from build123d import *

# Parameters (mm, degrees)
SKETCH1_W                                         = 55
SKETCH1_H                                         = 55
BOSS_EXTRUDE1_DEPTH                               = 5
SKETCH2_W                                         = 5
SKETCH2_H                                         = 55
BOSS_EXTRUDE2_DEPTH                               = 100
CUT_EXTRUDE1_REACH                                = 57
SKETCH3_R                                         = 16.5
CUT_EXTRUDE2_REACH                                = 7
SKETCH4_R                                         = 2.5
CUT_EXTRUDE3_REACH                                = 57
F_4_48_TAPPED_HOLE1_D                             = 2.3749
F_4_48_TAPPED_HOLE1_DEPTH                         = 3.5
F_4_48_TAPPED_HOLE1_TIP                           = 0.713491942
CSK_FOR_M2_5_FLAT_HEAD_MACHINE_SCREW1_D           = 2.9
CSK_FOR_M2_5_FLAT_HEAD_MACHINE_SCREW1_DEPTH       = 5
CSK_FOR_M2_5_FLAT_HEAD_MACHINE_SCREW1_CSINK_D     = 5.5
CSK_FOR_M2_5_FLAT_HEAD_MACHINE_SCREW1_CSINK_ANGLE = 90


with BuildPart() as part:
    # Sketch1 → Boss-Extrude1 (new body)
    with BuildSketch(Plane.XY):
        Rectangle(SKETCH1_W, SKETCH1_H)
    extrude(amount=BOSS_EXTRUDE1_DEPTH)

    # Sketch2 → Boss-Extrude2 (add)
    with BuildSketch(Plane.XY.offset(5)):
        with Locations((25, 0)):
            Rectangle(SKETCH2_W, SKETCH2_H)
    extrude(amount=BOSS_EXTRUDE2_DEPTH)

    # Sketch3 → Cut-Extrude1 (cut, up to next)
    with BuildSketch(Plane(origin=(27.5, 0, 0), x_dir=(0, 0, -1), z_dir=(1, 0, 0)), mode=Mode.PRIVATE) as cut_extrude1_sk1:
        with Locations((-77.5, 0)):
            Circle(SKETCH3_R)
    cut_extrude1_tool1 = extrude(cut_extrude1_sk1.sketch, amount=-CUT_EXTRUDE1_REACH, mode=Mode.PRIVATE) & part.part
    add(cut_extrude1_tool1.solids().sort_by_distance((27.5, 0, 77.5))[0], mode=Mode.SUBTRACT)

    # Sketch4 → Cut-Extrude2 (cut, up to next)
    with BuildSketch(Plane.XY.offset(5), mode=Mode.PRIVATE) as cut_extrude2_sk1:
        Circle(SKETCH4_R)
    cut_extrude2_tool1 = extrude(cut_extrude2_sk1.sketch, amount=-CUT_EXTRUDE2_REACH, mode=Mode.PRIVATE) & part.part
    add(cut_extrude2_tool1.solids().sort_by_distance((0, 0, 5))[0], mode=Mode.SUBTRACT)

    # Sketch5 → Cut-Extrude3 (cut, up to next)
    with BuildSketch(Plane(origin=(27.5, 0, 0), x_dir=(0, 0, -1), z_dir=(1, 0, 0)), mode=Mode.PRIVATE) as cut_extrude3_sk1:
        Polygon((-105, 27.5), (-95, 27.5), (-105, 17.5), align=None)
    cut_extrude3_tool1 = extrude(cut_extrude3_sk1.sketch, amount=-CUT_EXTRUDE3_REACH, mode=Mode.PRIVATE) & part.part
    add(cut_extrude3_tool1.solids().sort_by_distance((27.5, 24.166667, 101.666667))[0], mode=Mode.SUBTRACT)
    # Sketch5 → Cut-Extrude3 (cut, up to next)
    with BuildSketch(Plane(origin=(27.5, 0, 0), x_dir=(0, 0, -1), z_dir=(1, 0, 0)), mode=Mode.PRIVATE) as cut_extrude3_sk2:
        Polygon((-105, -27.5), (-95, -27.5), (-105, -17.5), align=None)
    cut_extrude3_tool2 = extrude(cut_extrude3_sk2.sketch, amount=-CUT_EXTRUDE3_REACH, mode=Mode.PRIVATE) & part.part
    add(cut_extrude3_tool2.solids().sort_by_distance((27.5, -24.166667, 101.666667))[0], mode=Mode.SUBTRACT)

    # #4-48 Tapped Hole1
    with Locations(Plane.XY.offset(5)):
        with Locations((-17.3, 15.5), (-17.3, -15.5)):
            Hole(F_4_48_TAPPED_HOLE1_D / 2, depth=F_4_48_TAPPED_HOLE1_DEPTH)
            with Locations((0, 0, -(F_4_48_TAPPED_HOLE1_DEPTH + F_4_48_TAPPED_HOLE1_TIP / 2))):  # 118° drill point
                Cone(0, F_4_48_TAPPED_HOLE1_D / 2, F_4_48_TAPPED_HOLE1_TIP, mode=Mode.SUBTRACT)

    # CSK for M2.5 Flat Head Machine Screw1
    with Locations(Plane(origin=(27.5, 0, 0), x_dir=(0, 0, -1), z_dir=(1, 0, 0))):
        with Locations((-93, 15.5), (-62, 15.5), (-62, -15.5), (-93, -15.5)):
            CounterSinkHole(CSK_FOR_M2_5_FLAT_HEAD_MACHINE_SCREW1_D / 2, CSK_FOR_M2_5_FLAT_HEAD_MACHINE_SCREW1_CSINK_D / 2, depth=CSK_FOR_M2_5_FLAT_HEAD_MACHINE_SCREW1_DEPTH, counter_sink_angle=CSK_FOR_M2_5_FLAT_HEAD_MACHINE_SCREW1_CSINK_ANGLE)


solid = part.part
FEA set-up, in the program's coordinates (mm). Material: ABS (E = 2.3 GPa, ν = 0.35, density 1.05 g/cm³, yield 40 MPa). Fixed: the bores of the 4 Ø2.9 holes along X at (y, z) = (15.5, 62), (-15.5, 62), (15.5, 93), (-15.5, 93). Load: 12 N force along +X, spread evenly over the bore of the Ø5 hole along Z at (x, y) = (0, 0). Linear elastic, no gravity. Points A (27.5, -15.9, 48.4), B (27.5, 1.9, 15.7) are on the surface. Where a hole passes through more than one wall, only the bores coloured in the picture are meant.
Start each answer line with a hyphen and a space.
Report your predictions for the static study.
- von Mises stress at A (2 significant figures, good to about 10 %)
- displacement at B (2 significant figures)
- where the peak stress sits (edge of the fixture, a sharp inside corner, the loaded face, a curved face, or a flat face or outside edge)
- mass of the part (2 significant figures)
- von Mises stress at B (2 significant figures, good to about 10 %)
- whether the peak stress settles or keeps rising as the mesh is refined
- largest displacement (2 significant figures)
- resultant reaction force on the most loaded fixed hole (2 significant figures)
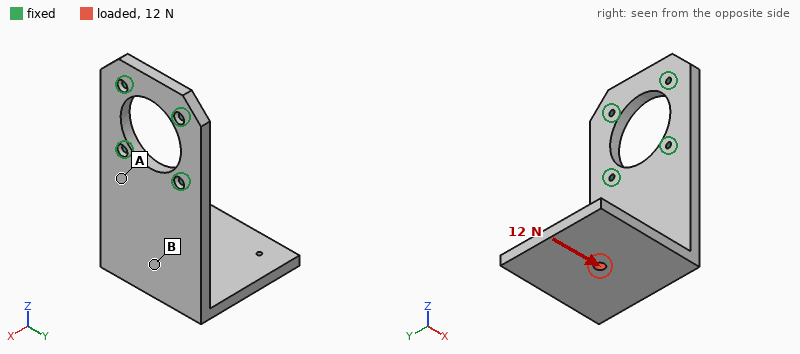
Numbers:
- 2.3 MPa
- 0.58 mm
- edge of the fixture
- 39 g
- 0.66 MPa
- keeps rising
- 1.3 mm
- 10 N
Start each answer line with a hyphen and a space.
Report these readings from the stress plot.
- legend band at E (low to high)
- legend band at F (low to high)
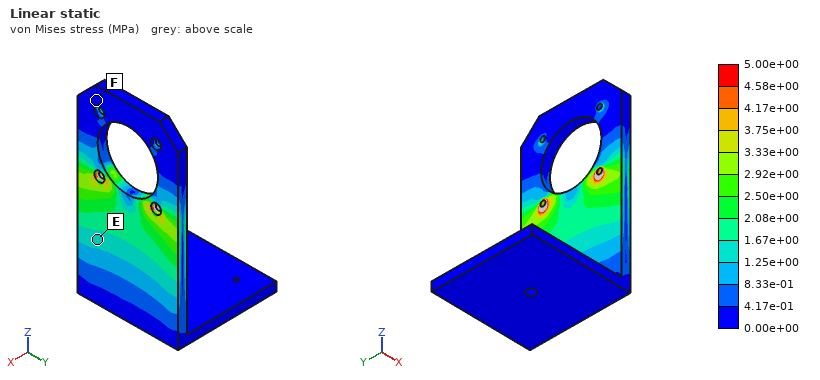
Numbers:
- 1.25e+00 to 1.67e+00 MPa
- 0.00e+00 to 4.17e-01 MPa
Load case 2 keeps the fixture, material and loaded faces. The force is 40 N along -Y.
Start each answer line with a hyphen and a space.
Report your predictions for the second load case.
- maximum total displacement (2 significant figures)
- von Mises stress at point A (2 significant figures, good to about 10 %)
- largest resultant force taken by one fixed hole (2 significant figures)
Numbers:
- 1.4 mm
- 2.8 MPa
- 60 N
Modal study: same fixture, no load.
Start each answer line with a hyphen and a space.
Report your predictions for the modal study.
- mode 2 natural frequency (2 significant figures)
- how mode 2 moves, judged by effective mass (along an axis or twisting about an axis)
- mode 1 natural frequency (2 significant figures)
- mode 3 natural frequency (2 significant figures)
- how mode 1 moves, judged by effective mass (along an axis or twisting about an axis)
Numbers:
- 240 Hz
- along Y
- 120 Hz
- 360 Hz
- along X
